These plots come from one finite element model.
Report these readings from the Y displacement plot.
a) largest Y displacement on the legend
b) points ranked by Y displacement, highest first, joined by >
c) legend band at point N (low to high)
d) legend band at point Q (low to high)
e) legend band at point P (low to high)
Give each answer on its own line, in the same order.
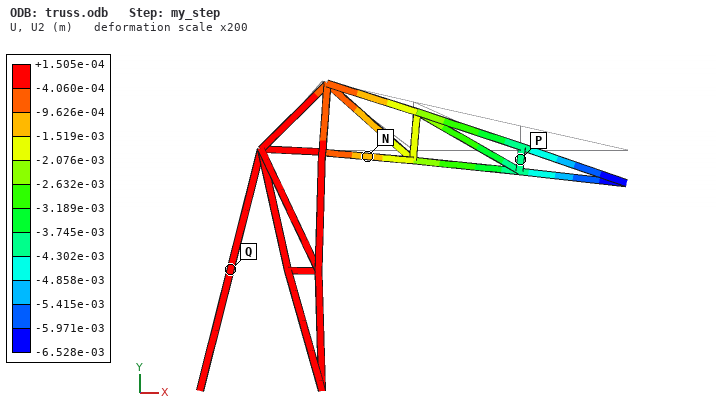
+1.505e-04 m
Q > N > P
-1.519e-03 to -9.626e-04 m
-4.060e-04 to +1.505e-04 m
-4.302e-03 to -3.745e-03 m
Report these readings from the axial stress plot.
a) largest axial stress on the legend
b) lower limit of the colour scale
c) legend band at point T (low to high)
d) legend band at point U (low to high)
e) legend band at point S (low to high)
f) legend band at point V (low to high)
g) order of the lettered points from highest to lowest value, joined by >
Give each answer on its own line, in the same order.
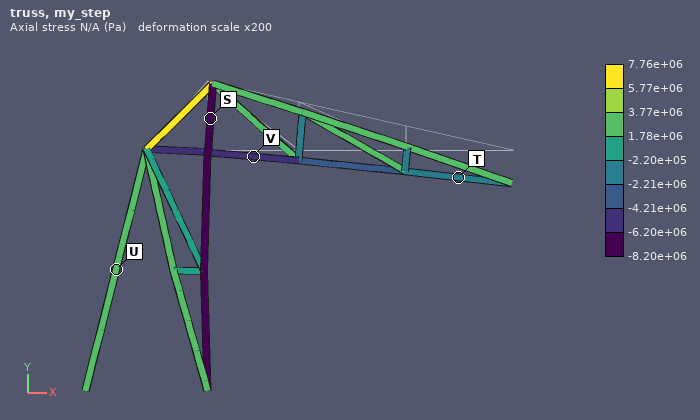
7.76e+06 Pa
-8.20e+06 Pa
-2.21e+06 to -2.20e+05 Pa
1.78e+06 to 3.77e+06 Pa
-8.20e+06 to -6.20e+06 Pa
-6.20e+06 to -4.21e+06 Pa
U > T > V > S
